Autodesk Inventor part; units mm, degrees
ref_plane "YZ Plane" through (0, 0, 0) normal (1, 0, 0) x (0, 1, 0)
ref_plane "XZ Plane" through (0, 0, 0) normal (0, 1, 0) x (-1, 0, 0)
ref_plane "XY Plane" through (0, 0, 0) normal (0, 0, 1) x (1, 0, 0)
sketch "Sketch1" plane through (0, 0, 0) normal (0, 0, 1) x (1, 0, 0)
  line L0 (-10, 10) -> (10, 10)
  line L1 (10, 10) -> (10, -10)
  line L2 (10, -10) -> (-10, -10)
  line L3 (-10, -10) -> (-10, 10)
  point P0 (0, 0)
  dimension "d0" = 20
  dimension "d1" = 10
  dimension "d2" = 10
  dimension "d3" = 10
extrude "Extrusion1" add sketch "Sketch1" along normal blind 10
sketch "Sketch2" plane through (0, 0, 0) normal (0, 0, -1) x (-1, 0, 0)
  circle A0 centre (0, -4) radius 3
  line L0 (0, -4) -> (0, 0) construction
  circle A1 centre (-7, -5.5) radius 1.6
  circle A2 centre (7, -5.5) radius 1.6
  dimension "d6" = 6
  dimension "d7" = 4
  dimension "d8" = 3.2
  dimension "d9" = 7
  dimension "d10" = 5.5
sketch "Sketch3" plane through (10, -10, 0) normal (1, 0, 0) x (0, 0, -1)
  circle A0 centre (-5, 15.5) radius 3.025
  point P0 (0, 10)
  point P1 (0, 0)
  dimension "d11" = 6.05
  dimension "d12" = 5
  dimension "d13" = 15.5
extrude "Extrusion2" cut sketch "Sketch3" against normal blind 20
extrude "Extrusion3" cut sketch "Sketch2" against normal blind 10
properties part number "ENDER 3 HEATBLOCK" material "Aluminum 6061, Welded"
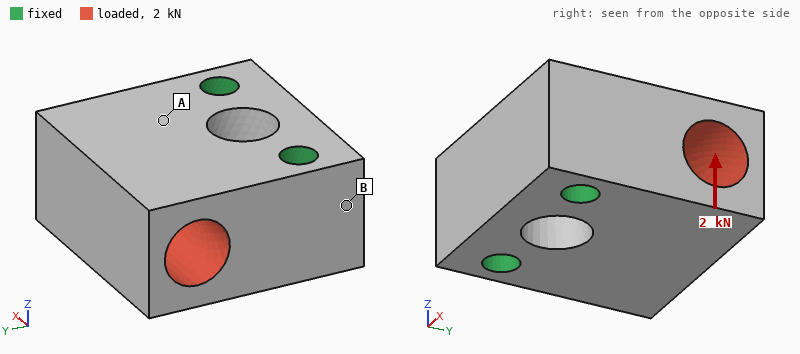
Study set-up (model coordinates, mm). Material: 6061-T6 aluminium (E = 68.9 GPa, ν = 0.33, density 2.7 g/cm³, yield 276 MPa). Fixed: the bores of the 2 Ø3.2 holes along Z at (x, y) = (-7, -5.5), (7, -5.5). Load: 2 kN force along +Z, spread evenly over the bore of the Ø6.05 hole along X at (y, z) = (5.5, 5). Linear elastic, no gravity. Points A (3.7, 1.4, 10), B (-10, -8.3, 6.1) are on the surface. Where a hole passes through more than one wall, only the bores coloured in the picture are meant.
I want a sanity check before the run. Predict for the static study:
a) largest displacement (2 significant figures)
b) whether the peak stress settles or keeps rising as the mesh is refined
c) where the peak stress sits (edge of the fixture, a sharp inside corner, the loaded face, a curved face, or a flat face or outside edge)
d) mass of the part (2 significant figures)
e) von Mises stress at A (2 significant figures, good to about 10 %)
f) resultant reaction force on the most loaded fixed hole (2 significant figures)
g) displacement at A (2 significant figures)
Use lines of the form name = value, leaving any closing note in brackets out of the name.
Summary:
largest displacement = 32 µm
whether the peak stress settles or keeps rising as the mesh is refined = keeps rising
where the peak stress sits = edge of the fixture
mass of the part = 8.0 g
von Mises stress at A = 49 MPa
resultant reaction force on the most loaded fixed hole = 1.0 kN
displacement at A = 11 µm
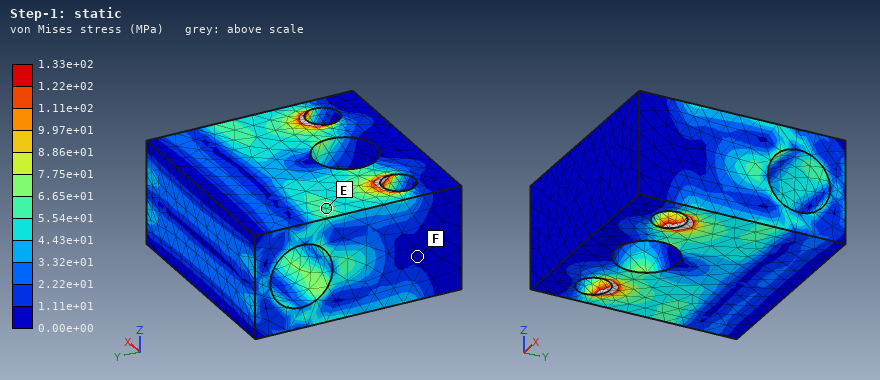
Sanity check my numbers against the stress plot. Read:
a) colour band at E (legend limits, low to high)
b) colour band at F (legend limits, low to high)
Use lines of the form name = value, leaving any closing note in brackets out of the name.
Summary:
colour band at E = 5.54e+01 to 6.65e+01 MPa
colour band at F = 0.00e+00 to 1.11e+01 MPa
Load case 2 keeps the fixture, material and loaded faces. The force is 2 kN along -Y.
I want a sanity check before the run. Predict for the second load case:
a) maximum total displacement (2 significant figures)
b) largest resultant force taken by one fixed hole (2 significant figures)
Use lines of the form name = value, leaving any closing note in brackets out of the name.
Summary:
maximum total displacement = 5.2 µm
largest resultant force taken by one fixed hole = 1.0 kN
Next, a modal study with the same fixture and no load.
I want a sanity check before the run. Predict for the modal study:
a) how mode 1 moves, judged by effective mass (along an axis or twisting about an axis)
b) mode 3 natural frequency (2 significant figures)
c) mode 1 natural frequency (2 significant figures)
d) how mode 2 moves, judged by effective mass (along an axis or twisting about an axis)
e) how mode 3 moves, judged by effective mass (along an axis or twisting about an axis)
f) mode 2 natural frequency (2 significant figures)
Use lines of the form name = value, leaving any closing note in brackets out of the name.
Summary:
how mode 1 moves, judged by effective mass = along Z
mode 3 natural frequency = 41 kHz
mode 1 natural frequency = 25 kHz
how mode 2 moves, judged by effective mass = along X
how mode 3 moves, judged by effective mass = twisting about Y
mode 2 natural frequency = 39 kHz
